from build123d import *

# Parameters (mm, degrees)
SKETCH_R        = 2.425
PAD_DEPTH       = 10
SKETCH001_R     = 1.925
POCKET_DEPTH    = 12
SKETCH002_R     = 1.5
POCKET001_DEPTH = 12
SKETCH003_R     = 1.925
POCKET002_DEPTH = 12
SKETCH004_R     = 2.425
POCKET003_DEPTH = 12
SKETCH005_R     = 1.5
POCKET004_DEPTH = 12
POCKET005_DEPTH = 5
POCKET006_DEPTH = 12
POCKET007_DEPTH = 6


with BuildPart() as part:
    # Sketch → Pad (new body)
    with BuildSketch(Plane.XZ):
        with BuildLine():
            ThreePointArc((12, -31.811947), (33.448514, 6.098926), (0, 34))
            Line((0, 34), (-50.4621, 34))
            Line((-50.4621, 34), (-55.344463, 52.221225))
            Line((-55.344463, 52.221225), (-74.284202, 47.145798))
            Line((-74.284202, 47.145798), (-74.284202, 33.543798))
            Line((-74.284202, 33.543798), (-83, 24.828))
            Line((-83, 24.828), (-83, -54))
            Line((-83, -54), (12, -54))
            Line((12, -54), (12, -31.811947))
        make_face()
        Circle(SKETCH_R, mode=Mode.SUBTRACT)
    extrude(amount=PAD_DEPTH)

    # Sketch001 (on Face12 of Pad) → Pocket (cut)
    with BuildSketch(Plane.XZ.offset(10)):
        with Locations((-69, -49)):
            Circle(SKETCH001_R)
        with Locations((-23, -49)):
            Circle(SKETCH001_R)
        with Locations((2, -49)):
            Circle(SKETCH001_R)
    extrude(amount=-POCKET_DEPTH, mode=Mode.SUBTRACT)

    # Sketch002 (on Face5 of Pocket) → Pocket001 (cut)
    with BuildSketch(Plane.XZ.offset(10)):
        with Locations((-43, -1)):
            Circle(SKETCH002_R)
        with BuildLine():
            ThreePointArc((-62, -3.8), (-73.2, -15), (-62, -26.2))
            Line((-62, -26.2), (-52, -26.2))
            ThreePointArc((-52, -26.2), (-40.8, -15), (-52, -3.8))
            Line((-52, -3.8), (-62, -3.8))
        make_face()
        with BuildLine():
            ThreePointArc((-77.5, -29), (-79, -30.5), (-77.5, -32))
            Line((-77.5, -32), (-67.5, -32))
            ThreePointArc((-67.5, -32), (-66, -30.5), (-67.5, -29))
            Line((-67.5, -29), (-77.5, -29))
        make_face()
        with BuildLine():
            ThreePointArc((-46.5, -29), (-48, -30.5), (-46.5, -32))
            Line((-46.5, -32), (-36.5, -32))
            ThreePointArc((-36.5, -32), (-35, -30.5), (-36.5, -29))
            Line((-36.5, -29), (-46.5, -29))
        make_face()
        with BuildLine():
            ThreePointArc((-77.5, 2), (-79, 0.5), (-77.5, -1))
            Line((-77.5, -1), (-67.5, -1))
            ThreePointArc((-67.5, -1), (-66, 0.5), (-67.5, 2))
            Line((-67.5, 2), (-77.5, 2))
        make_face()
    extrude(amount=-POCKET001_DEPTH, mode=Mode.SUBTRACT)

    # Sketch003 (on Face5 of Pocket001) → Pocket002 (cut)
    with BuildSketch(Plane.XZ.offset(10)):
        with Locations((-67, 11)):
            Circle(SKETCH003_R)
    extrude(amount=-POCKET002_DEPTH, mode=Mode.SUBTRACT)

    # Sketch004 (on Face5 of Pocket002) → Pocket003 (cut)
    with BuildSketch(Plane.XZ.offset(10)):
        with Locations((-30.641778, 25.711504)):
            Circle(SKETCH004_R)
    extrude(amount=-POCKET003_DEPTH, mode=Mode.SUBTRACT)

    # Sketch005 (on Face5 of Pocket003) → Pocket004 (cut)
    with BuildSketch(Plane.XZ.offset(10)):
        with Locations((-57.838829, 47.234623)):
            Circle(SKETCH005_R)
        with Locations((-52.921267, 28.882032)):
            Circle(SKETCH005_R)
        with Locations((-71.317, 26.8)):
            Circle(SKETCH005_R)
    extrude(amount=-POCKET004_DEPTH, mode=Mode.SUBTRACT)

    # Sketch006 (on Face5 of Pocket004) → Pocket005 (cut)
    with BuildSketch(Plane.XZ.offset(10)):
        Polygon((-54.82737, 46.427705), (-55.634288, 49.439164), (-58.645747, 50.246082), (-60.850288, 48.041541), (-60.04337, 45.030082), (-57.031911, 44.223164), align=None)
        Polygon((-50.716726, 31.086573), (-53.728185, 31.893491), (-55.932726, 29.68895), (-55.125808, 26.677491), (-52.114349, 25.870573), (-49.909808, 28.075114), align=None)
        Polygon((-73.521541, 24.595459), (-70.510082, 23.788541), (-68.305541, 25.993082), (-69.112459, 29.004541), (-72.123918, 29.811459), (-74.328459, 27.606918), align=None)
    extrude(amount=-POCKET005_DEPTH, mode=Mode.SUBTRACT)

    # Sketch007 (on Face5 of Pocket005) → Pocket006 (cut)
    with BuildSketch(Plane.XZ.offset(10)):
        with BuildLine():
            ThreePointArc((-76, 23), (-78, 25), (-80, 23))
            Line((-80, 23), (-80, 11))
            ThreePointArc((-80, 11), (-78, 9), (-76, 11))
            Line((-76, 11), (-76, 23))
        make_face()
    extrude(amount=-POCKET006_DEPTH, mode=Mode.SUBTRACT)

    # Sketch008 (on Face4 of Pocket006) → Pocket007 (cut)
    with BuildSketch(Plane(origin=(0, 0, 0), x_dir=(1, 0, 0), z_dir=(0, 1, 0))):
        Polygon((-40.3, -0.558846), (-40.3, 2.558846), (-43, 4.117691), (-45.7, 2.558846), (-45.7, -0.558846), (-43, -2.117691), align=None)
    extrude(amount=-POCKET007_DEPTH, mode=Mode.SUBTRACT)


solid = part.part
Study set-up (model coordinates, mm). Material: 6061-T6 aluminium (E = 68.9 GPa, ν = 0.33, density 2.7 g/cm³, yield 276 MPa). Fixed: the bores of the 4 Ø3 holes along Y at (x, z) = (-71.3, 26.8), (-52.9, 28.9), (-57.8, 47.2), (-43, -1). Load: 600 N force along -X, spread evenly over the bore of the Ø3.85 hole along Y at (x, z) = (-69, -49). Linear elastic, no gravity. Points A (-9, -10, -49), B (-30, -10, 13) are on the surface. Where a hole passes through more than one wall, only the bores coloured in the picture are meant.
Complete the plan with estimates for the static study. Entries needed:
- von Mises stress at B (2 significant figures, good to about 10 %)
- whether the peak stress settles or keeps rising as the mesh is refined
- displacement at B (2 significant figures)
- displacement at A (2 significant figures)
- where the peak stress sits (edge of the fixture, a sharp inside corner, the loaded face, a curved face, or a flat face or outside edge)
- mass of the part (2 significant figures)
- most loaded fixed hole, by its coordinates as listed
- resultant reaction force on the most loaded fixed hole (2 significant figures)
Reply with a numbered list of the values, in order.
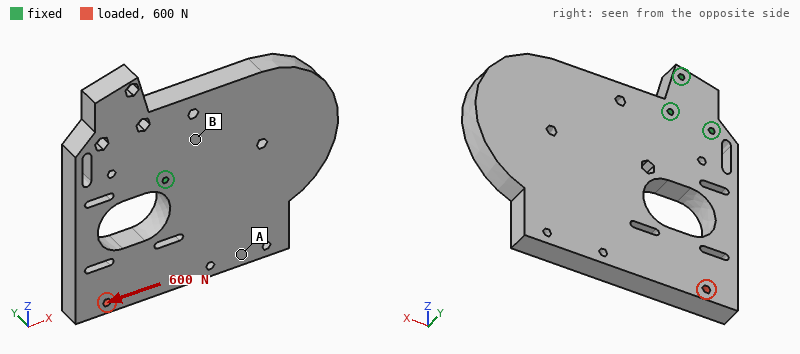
1. 3.8 MPa
2. keeps rising
3. 6.0 µm
4. 18 µm
5. edge of the fixture
6. 240 g
7. (-43, -1)
8. 1.1 kN
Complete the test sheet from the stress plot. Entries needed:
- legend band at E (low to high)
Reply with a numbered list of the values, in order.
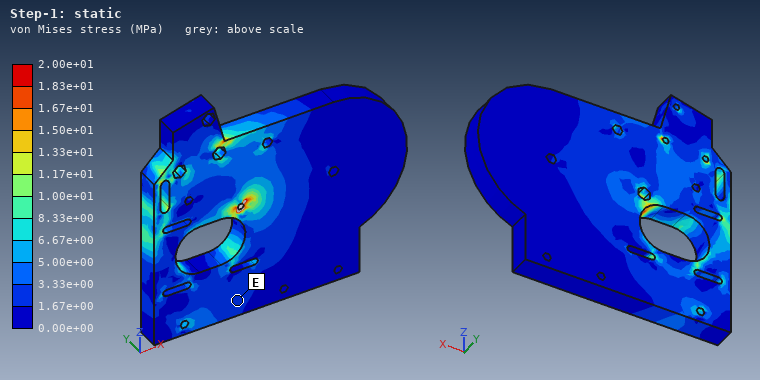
1. 1.67e+00 to 3.33e+00 MPa
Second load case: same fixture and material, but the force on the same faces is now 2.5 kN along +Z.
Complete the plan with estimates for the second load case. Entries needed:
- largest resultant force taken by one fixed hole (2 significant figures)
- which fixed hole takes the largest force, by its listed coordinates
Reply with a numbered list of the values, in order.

1. 1.1 kN
2. (-71.3, 26.8)
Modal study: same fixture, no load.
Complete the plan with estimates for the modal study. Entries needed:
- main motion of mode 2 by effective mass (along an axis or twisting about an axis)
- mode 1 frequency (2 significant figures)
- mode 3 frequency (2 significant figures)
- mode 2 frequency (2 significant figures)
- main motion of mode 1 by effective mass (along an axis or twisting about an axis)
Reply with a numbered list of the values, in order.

1. along Y
2. 930 Hz
3. 2700 Hz
4. 1400 Hz
5. along Y
